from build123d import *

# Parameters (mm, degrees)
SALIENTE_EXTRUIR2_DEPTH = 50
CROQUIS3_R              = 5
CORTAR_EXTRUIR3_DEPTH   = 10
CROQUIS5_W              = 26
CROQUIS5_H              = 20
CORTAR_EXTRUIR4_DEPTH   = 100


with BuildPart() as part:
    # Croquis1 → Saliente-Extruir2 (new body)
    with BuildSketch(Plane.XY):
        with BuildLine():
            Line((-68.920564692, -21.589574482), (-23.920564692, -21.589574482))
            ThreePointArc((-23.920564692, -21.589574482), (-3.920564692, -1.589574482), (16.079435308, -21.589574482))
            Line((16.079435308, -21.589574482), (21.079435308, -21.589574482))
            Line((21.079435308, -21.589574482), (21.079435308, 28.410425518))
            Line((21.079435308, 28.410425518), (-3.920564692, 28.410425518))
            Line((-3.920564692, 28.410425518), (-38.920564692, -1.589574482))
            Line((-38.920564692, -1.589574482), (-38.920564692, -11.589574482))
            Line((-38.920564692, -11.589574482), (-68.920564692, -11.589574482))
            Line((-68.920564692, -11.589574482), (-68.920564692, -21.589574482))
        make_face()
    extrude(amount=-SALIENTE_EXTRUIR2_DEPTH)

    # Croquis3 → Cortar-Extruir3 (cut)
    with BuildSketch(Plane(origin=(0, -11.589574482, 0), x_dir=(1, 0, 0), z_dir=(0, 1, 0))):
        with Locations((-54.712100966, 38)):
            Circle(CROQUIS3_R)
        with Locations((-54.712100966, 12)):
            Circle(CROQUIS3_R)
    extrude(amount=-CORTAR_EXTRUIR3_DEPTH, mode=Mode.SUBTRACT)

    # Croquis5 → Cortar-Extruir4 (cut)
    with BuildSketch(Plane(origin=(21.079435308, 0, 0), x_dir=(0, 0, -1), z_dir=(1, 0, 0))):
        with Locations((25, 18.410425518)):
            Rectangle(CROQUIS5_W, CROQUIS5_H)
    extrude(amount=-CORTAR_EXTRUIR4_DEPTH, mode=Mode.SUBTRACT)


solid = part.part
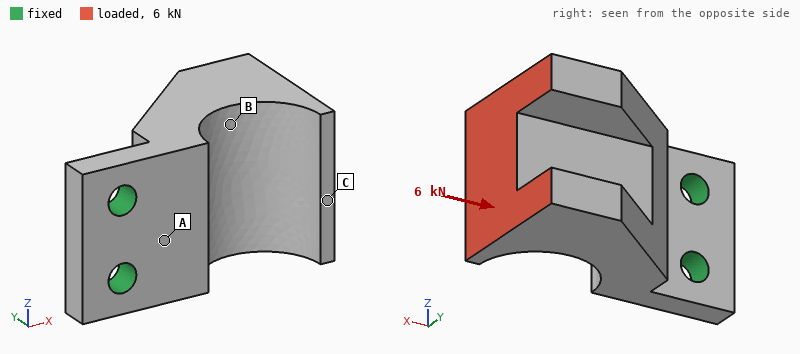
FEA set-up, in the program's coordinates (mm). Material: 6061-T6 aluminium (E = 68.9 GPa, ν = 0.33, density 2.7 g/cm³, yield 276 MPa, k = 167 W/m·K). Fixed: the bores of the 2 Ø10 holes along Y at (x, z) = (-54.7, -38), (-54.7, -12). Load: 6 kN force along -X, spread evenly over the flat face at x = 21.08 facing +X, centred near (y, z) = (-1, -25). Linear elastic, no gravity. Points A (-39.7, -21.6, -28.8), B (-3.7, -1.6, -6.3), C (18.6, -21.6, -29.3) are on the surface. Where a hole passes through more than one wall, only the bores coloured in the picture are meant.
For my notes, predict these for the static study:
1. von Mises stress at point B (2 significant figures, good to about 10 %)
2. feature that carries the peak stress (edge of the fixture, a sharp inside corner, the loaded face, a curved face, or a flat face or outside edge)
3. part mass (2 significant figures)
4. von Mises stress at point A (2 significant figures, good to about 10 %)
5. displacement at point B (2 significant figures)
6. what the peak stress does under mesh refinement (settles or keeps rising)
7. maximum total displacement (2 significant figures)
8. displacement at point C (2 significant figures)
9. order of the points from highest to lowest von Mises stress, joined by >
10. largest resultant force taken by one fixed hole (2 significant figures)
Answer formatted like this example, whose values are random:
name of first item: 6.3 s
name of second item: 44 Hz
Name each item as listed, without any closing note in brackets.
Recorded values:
von Mises stress at point B: 28 MPa
feature that carries the peak stress: edge of the fixture
part mass: 230 g
von Mises stress at point A: 83 MPa
displacement at point B: 0.25 mm
what the peak stress does under mesh refinement: keeps rising
maximum total displacement: 0.45 mm
displacement at point C: 0.35 mm
order of the points from highest to lowest von Mises stress, joined by >: A > B > C
largest resultant force taken by one fixed hole: 3.0 kN
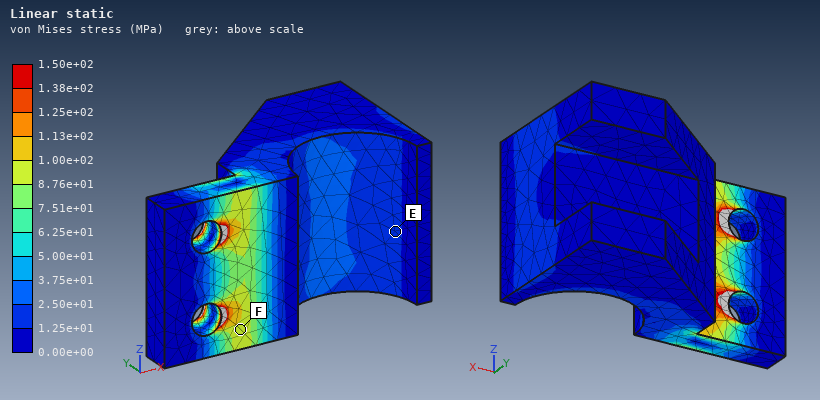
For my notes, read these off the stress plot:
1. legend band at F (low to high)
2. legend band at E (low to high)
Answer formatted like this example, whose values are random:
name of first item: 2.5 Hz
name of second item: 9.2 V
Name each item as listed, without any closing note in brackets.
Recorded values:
legend band at F: 8.76e+01 to 1.00e+02 MPa
legend band at E: 1.25e+01 to 2.50e+01 MPa
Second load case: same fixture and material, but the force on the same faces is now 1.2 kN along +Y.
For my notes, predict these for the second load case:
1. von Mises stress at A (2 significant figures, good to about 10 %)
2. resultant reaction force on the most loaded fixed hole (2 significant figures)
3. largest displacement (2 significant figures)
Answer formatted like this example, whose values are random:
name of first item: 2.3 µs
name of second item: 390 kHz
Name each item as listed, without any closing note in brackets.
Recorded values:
von Mises stress at A: 71 MPa
resultant reaction force on the most loaded fixed hole: 610 N
largest displacement: 0.43 mm
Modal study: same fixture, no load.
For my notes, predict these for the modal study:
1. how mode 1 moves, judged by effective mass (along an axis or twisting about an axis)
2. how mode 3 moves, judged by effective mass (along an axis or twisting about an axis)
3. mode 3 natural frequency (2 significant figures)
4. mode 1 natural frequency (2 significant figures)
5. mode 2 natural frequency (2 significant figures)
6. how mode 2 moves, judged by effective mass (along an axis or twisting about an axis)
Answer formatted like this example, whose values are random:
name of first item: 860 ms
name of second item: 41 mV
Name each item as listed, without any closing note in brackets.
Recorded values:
how mode 1 moves, judged by effective mass: along Y
how mode 3 moves, judged by effective mass: twisting about X
mode 3 natural frequency: 3200 Hz
mode 1 natural frequency: 950 Hz
mode 2 natural frequency: 2800 Hz
how mode 2 moves, judged by effective mass: along Z
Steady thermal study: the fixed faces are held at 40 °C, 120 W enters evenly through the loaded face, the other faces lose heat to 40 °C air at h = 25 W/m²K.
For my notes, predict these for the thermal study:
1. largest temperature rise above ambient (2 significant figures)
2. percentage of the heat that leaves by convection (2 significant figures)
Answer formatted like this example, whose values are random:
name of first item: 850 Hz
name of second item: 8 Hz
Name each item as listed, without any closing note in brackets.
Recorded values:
largest temperature rise above ambient: 74 K
percentage of the heat that leaves by convection: 13 %
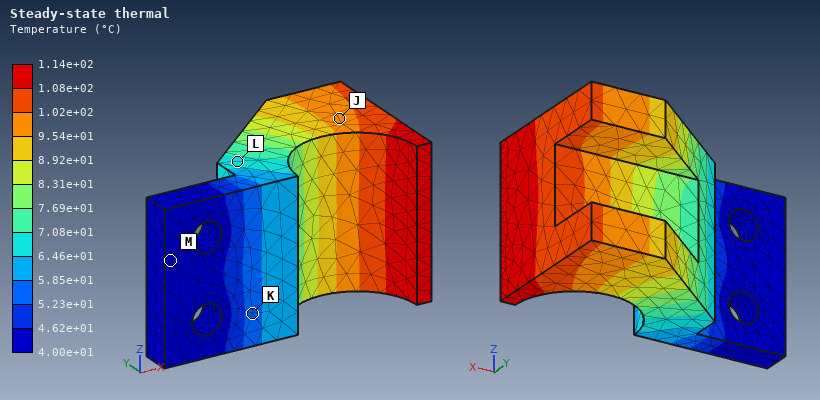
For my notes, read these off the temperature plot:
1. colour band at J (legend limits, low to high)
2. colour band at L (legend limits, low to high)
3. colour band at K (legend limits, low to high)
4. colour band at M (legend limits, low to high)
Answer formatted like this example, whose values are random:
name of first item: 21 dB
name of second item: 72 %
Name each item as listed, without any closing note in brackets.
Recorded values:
colour band at J: 9.54e+01 to 1.02e+02 °C
colour band at L: 6.46e+01 to 7.08e+01 °C
colour band at K: 5.23e+01 to 5.85e+01 °C
colour band at M: 4.00e+01 to 4.62e+01 °C
